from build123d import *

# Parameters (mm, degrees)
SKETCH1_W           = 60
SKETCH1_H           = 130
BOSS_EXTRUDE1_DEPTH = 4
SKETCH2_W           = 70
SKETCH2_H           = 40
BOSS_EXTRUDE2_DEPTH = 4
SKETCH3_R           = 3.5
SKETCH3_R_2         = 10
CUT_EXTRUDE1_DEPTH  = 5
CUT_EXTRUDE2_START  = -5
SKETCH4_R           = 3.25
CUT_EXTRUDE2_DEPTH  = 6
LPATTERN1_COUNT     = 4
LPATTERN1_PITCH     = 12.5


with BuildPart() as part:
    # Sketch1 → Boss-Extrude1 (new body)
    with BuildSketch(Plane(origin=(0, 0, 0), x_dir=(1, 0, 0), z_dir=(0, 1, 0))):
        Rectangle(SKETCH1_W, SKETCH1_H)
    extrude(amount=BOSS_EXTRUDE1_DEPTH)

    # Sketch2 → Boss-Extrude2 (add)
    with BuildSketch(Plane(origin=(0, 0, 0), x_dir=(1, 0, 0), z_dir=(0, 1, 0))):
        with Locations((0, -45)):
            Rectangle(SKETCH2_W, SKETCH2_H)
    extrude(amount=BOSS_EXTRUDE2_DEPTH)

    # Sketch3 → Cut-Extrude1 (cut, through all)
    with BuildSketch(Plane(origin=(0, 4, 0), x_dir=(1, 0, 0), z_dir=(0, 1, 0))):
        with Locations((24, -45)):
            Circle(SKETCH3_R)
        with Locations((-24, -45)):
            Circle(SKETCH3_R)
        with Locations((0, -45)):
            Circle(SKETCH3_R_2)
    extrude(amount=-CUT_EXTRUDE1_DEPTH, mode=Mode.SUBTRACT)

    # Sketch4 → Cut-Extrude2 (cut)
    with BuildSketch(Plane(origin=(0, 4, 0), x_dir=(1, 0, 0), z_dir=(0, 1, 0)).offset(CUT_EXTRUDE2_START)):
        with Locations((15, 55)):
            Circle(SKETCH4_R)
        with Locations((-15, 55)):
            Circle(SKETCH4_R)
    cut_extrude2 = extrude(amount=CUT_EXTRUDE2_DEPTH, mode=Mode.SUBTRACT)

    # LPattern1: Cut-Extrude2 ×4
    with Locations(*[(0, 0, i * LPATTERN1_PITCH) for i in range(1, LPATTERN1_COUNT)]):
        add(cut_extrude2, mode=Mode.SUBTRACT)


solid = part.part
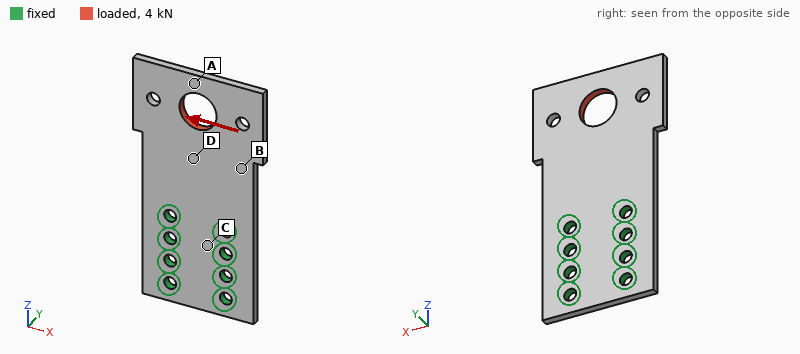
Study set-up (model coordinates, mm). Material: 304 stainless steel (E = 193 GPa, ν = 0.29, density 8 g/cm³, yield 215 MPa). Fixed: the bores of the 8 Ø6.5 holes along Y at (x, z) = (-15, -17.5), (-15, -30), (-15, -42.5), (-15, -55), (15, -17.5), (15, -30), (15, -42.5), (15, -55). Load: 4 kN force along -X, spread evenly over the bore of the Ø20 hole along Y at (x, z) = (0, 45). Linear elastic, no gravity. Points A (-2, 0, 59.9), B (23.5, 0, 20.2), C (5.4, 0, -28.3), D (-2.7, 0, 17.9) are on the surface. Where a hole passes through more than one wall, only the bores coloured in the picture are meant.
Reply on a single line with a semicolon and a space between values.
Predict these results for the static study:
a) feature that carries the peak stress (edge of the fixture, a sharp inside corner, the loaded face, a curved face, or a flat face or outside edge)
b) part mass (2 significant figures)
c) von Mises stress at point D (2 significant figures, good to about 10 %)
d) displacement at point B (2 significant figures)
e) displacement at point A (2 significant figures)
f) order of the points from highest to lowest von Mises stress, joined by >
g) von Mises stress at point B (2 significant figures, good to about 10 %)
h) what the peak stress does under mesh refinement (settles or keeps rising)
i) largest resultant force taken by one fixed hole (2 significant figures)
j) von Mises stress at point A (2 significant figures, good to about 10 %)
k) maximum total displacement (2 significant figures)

edge of the fixture; 240 g; 52 MPa; 28 µm; 63 µm; D > B > A > C; 34 MPa; keeps rising; 5.3 kN; 22 MPa; 73 µm
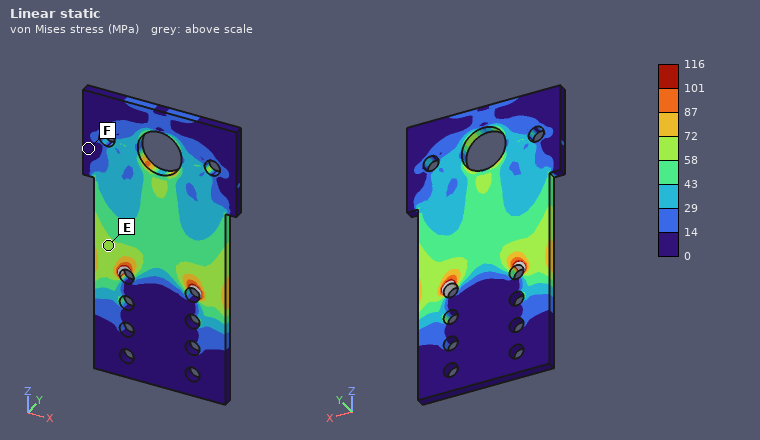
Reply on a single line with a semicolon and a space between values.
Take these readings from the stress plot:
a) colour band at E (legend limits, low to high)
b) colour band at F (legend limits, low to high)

58 to 72 MPa; 0 to 14 MPa
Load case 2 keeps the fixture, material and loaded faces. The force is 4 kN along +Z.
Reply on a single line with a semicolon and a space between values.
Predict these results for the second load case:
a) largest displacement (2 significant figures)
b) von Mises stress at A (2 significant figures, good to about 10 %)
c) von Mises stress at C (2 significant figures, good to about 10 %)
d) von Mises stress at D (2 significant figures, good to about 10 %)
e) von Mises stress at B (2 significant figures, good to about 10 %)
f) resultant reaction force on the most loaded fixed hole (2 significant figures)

10 µm; 18 MPa; 4.7 MPa; 19 MPa; 15 MPa; 1.5 kN
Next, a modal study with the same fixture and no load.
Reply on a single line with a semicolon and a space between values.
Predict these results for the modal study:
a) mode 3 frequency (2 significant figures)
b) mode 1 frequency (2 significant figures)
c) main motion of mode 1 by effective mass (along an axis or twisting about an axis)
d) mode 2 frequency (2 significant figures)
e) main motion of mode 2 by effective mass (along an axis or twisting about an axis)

2800 Hz; 480 Hz; along Y; 1200 Hz; twisting about Z
